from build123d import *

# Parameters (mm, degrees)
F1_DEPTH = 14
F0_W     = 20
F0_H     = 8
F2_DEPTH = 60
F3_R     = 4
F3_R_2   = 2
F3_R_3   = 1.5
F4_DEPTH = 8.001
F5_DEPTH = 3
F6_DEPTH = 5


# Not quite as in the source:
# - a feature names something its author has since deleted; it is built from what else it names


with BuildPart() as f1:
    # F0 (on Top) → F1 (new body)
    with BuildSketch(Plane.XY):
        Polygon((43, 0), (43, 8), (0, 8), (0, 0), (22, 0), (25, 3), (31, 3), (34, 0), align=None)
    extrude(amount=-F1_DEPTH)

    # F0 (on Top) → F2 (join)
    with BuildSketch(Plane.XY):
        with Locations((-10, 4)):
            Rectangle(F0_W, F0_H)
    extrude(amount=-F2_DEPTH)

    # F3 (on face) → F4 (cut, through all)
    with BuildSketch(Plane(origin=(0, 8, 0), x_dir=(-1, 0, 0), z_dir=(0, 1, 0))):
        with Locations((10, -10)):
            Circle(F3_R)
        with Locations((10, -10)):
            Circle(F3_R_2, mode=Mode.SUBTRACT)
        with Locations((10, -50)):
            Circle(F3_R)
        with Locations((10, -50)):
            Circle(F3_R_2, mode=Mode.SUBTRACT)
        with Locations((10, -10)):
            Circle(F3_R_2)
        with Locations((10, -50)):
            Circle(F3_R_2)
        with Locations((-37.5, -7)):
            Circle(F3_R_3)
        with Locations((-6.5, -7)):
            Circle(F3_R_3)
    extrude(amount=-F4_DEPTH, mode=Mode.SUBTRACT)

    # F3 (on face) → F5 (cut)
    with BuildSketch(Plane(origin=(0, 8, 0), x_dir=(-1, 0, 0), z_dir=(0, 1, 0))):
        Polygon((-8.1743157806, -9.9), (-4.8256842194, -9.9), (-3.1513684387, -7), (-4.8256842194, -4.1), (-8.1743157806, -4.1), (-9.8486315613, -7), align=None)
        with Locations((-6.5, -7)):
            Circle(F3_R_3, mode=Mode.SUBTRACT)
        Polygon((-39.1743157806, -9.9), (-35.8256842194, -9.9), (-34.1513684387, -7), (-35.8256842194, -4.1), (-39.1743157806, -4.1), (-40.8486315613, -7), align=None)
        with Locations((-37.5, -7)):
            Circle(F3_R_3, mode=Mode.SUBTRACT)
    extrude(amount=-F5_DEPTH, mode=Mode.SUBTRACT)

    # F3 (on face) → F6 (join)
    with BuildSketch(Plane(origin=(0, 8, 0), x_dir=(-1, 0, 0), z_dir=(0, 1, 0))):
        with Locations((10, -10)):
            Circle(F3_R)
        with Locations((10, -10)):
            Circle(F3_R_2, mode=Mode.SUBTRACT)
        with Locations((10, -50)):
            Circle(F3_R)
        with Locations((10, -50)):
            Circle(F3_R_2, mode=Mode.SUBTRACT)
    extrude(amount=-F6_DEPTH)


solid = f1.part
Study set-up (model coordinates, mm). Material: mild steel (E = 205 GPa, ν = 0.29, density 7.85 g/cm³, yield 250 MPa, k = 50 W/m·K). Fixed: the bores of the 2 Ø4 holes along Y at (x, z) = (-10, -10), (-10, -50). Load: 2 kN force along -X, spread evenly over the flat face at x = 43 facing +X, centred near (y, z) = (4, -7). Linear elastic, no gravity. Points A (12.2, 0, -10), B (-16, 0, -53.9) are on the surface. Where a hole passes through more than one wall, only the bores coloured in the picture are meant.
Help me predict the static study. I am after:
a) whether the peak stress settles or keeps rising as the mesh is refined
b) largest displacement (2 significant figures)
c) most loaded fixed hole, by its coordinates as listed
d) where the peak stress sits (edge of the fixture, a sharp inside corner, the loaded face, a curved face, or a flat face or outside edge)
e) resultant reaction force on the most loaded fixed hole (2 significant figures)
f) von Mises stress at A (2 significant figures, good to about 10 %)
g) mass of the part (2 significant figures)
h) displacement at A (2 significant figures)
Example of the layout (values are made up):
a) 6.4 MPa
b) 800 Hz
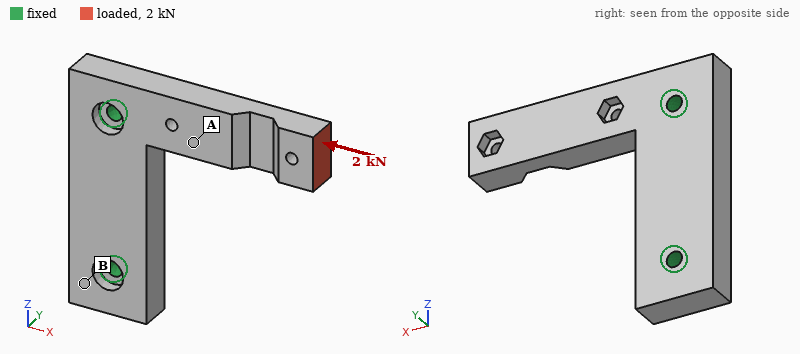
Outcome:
a) keeps rising
b) 26 µm
c) (-10, -10)
d) edge of the fixture
e) 2.1 kN
f) 18 MPa
g) 100 g
h) 5.6 µm
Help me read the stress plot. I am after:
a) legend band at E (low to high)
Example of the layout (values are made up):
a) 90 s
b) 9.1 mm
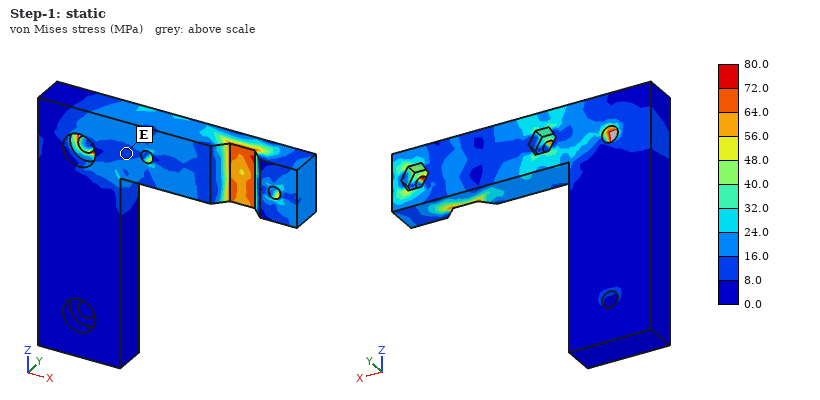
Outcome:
a) 8.0 to 16.0 MPa
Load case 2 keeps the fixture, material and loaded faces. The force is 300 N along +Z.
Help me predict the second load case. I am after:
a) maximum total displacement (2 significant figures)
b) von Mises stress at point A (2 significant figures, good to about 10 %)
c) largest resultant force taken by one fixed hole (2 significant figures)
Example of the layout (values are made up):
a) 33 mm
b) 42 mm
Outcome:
a) 47 µm
b) 17 MPa
c) 380 N
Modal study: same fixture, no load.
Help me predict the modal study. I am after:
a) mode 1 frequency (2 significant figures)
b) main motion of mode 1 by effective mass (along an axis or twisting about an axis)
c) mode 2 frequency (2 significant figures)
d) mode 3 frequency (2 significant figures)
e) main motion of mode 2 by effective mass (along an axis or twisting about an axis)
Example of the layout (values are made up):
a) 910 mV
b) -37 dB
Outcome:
a) 2100 Hz
b) along Y
c) 4100 Hz
d) 10 kHz
e) along Z
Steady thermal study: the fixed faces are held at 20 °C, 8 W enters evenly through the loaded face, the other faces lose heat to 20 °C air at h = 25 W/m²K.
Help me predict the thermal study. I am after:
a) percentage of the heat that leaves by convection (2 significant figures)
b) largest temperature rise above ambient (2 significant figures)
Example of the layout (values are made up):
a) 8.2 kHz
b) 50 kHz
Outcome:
a) 28 %
b) 76 K
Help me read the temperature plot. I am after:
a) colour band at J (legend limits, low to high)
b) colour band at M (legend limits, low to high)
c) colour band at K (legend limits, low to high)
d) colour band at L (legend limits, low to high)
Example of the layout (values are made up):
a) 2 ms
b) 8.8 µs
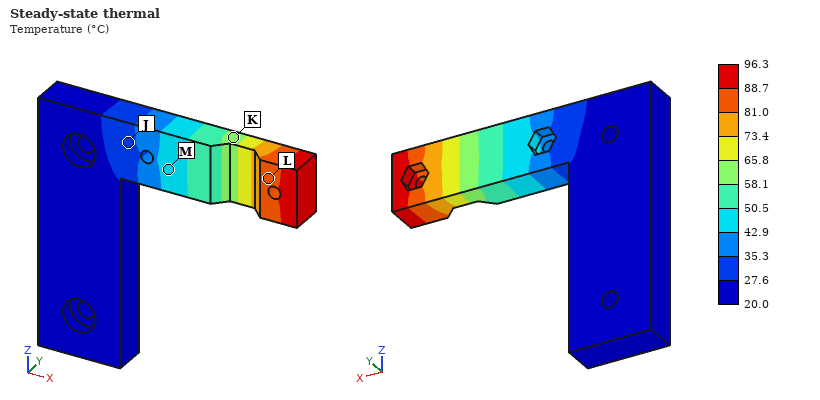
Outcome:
a) 27.6 to 35.3 °C
b) 42.9 to 50.5 °C
c) 58.1 to 65.8 °C
d) 81.0 to 88.7 °C
